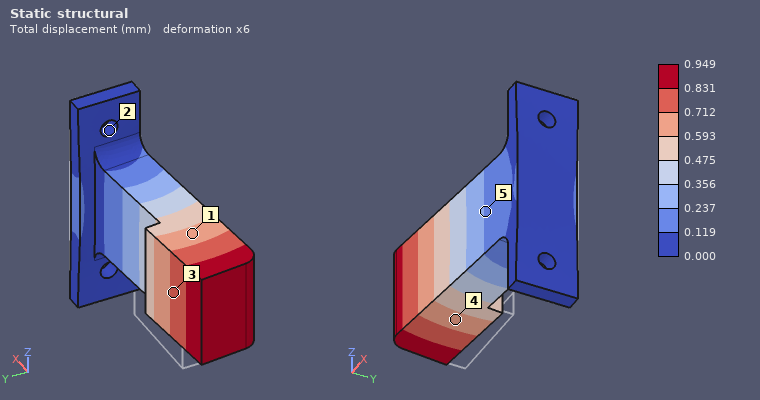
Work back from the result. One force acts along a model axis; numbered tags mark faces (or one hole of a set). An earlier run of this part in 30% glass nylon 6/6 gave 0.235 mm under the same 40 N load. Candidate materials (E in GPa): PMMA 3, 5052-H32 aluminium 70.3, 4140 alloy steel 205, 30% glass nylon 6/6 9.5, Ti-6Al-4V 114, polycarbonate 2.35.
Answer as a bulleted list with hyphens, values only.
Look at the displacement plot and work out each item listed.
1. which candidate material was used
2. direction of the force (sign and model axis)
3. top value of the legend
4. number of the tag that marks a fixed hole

- polycarbonate
- -Y
- 0.949 mm
- 2
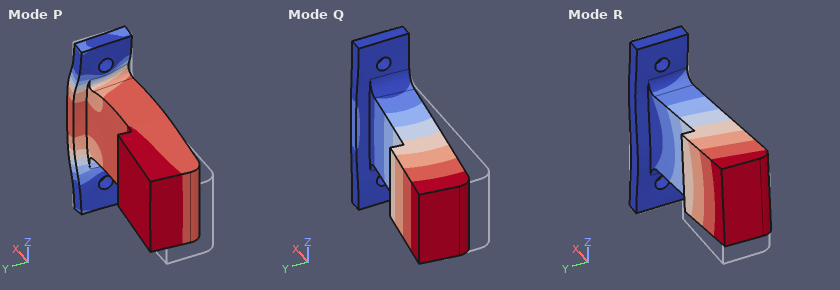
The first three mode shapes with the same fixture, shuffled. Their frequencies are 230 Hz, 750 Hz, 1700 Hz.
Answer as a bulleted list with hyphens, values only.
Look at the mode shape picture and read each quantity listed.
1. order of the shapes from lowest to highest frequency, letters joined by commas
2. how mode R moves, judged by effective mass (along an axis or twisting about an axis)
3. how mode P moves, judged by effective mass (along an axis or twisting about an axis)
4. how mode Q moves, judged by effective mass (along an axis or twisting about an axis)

- Q, R, P
- along Z
- along X
- along Y
